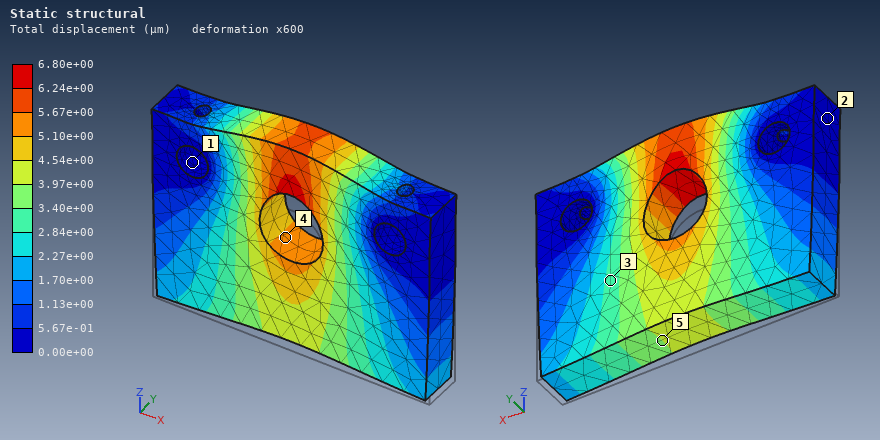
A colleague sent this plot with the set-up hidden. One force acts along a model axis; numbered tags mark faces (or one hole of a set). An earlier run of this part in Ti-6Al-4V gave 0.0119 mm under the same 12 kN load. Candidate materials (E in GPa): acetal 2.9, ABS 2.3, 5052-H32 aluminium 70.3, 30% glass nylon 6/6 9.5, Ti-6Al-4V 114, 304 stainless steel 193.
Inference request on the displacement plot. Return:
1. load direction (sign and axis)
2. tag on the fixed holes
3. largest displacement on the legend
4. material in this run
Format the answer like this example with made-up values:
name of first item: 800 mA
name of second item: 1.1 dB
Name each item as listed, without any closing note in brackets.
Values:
load direction: +Z
tag on the fixed holes: 1
largest displacement on the legend: 6.80e+00 µm
material in this run: 304 stainless steel
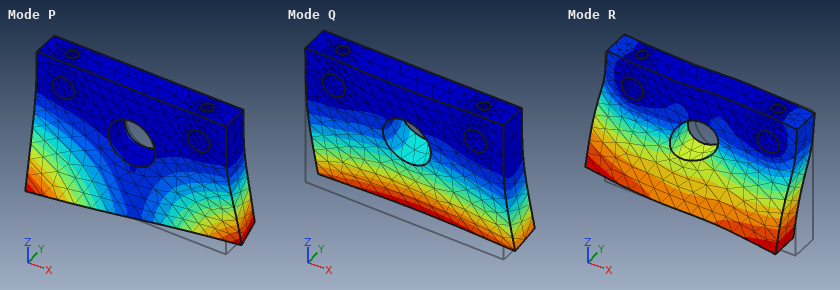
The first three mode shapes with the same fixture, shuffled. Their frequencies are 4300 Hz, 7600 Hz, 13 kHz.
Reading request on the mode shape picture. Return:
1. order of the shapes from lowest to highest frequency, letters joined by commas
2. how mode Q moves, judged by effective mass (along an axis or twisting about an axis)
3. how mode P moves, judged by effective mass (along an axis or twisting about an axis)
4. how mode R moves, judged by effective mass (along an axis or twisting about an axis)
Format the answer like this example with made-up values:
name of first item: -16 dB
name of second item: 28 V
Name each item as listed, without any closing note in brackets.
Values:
order of the shapes from lowest to highest frequency, letters joined by commas: Q, P, R
how mode Q moves, judged by effective mass: along Y
how mode P moves, judged by effective mass: twisting about Z
how mode R moves, judged by effective mass: along X
